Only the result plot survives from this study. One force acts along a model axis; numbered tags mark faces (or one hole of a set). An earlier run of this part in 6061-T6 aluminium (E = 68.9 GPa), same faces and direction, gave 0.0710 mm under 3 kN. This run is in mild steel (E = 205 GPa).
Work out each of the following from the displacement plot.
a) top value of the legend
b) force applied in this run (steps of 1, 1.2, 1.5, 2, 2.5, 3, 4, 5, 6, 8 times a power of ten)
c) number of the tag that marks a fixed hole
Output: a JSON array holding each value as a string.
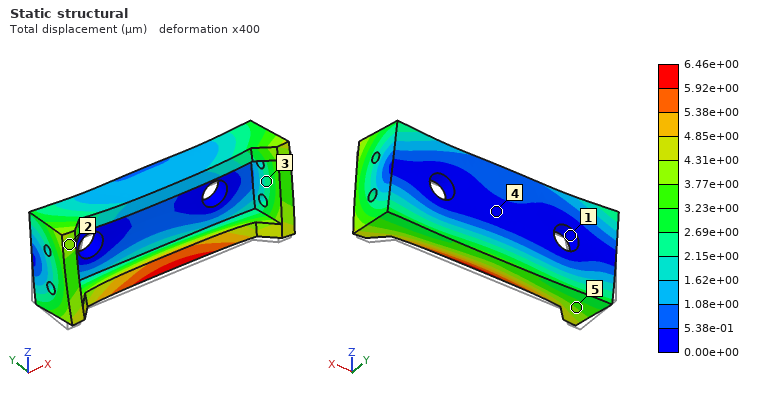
["6.46e+00 µm", "800 N", "1"]
